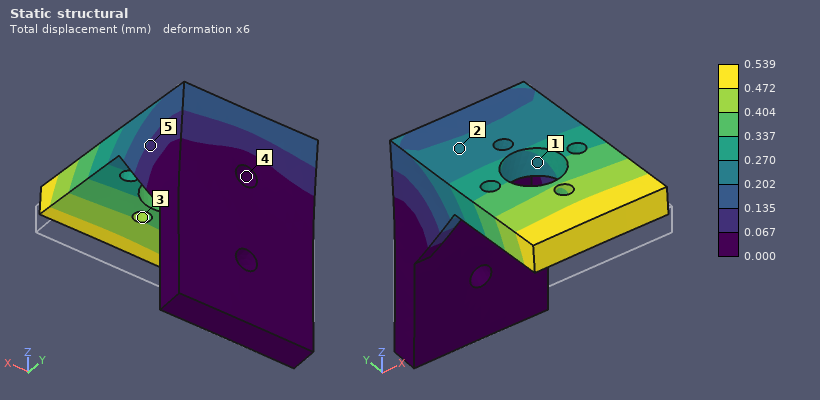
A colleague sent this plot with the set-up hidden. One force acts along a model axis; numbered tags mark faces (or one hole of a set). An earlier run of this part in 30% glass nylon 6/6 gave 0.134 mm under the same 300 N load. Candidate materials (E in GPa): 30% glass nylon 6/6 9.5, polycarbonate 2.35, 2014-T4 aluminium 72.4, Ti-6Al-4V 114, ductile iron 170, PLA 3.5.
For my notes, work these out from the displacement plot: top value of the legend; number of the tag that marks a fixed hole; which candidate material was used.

0.539 mm
4
polycarbonate
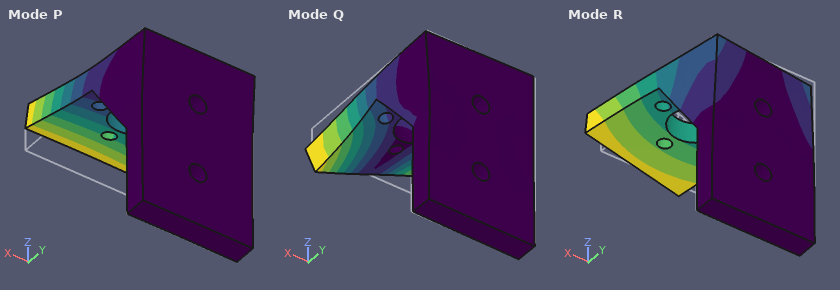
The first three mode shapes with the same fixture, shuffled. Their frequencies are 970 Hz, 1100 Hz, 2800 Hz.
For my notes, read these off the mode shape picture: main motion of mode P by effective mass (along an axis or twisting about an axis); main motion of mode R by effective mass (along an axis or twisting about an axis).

along Z
along X
